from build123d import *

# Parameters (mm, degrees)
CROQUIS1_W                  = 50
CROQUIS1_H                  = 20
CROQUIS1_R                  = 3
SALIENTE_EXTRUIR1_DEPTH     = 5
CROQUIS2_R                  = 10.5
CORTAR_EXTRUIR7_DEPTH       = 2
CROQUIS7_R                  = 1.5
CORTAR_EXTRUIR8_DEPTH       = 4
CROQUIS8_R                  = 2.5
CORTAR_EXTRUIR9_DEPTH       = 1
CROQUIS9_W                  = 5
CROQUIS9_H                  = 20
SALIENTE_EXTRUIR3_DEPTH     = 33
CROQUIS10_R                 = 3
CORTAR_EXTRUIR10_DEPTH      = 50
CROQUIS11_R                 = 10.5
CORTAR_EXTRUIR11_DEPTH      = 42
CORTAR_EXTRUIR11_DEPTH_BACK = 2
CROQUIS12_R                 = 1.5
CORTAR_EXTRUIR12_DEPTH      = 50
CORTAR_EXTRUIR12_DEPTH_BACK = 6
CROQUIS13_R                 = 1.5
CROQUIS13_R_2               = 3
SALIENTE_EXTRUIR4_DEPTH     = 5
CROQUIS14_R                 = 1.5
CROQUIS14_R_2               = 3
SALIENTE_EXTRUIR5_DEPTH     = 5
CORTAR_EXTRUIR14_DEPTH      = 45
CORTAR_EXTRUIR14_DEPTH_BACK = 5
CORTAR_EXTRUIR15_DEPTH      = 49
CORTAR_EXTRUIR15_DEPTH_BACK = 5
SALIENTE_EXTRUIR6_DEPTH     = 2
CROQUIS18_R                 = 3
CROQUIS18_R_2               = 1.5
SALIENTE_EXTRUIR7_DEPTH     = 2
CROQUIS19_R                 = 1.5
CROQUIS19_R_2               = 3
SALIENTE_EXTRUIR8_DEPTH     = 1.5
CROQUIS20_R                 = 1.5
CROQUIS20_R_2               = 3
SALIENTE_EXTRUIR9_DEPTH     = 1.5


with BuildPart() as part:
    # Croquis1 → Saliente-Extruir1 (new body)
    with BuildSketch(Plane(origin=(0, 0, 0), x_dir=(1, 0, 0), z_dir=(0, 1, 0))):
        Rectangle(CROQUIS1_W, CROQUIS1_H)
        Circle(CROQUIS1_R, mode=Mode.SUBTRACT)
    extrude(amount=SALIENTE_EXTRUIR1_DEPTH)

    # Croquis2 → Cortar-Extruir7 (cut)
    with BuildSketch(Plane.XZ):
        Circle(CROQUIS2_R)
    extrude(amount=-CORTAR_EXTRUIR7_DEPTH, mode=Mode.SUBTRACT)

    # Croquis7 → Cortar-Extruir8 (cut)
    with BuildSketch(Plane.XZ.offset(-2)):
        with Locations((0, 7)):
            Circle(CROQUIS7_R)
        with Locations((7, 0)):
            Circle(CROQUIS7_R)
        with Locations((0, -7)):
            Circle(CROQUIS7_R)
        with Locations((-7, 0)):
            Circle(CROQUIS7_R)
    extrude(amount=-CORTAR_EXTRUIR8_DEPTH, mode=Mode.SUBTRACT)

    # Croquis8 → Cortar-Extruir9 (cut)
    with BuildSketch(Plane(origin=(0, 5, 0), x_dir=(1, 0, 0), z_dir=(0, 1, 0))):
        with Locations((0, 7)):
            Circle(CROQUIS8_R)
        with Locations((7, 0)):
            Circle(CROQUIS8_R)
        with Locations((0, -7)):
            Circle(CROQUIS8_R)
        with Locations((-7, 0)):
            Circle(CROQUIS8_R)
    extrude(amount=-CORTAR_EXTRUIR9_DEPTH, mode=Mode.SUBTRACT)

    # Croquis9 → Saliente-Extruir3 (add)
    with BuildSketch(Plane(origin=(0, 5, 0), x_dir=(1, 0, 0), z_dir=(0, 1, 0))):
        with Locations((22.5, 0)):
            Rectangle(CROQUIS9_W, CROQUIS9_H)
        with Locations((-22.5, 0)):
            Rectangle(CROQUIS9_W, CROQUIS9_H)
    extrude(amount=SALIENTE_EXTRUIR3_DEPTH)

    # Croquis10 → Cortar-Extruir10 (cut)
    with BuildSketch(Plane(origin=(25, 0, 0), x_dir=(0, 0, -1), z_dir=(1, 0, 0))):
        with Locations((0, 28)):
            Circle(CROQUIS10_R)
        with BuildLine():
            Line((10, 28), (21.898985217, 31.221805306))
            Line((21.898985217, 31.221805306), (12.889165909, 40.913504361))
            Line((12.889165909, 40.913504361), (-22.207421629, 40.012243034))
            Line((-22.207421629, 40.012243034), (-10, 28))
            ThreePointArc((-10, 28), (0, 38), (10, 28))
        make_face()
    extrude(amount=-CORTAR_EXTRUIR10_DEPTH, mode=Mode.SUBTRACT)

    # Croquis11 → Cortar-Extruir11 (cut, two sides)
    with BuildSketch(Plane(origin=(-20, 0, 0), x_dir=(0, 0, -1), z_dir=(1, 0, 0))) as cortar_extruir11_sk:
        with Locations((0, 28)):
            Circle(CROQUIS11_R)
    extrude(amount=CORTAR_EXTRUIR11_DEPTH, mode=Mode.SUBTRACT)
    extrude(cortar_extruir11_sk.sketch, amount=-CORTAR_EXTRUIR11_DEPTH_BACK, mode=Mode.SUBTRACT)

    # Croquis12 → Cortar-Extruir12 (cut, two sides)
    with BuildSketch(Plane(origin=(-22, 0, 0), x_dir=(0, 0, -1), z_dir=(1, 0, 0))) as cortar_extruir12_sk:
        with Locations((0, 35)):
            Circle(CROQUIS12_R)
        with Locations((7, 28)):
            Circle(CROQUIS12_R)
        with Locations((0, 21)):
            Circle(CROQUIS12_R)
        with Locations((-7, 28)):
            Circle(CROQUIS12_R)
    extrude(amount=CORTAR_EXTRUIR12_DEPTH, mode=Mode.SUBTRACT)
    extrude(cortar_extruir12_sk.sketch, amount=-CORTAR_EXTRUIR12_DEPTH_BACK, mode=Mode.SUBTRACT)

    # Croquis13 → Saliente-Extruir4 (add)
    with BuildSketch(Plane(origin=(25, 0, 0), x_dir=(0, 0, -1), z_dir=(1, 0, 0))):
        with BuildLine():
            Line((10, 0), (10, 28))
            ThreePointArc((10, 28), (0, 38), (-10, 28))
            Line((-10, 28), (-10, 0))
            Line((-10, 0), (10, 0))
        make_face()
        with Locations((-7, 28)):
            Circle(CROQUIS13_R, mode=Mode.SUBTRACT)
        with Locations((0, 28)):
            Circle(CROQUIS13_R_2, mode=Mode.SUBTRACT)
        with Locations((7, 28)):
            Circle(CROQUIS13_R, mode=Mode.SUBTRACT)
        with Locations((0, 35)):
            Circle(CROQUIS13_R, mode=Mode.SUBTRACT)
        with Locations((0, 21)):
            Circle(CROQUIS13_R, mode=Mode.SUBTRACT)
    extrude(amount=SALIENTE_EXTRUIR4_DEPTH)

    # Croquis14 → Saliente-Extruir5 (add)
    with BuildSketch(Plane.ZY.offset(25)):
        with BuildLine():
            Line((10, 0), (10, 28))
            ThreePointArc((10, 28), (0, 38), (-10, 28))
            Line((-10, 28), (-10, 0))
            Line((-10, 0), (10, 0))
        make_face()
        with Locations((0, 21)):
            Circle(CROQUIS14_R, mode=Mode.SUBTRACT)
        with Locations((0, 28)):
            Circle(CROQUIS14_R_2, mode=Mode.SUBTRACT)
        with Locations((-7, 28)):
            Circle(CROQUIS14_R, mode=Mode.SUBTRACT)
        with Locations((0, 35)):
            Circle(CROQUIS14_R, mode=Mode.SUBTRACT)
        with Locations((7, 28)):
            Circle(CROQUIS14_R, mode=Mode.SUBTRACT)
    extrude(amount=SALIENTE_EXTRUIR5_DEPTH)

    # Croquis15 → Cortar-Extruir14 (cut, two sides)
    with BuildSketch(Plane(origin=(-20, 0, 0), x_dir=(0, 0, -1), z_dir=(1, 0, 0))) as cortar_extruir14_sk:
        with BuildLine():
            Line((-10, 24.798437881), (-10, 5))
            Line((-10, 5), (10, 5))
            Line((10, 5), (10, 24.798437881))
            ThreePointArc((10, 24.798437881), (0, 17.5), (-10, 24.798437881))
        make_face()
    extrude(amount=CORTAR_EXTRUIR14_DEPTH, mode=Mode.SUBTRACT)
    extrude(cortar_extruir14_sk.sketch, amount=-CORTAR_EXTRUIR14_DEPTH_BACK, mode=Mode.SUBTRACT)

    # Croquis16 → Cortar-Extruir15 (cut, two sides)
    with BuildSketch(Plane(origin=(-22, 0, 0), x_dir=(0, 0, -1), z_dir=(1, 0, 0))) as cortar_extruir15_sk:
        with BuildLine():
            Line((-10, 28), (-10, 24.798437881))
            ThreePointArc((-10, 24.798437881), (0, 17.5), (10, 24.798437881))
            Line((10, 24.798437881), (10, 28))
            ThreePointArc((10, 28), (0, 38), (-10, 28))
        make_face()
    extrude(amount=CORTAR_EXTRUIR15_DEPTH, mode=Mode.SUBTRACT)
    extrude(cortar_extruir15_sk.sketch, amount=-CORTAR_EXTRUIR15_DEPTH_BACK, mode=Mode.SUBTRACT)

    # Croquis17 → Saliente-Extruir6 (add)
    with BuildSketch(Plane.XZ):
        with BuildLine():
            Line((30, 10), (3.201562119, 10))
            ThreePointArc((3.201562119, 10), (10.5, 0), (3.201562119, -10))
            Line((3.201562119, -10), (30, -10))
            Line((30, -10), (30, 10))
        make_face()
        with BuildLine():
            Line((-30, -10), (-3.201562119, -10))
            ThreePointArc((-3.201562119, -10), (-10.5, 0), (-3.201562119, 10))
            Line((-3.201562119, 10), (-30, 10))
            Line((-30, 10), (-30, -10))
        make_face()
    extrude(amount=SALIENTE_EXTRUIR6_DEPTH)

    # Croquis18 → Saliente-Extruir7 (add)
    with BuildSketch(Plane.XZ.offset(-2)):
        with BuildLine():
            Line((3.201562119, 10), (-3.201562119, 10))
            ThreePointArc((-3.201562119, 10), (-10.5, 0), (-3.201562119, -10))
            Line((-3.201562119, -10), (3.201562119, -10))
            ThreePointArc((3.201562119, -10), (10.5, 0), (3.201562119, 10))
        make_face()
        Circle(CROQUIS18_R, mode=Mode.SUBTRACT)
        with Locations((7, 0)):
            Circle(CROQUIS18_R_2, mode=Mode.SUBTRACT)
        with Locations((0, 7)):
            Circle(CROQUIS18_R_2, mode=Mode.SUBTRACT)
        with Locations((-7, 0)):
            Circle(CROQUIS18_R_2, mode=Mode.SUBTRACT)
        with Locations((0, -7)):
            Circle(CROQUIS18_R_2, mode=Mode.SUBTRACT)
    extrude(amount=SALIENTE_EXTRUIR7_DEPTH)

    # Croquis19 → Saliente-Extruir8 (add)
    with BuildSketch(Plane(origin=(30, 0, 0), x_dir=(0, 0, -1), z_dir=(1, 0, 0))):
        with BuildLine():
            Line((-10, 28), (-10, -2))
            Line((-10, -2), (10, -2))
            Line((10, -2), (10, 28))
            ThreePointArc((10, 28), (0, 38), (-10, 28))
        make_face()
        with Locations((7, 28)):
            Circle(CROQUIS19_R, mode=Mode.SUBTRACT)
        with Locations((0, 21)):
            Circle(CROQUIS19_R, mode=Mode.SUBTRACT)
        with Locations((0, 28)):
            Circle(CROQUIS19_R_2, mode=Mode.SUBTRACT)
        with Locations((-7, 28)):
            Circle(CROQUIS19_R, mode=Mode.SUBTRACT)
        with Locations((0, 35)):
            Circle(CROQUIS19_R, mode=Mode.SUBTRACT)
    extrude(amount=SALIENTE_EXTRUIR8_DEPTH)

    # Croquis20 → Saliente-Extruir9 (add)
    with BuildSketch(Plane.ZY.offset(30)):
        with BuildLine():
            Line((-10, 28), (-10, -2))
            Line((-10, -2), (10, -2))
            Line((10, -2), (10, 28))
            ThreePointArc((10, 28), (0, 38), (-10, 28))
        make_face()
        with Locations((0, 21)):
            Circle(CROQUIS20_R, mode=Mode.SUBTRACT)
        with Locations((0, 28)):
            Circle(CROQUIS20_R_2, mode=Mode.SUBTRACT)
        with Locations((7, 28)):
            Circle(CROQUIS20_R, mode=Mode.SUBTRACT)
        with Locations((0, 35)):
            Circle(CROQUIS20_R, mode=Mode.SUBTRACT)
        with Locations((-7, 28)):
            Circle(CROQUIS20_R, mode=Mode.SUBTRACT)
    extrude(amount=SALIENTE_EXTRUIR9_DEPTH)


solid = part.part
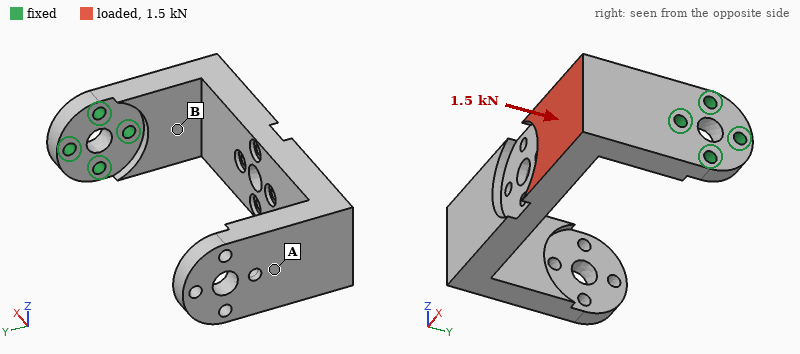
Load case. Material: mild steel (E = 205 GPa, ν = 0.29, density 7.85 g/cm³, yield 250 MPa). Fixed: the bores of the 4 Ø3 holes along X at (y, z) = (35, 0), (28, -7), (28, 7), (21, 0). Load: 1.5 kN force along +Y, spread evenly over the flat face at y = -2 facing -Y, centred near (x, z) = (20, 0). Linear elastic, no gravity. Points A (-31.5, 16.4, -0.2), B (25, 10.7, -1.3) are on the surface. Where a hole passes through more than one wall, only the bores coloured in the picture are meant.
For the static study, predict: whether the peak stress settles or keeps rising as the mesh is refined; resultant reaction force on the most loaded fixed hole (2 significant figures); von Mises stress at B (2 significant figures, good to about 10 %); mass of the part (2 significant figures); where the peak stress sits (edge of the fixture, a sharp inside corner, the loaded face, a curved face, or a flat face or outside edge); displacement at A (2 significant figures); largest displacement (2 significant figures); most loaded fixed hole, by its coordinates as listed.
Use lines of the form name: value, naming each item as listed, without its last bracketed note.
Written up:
whether the peak stress settles or keeps rising as the mesh is refined: keeps rising
resultant reaction force on the most loaded fixed hole: 1.1 kN
von Mises stress at B: 87 MPa
mass of the part: 110 g
where the peak stress sits: edge of the fixture
displacement at A: 0.24 mm
largest displacement: 0.26 mm
most loaded fixed hole, by its coordinates as listed: (21, 0)
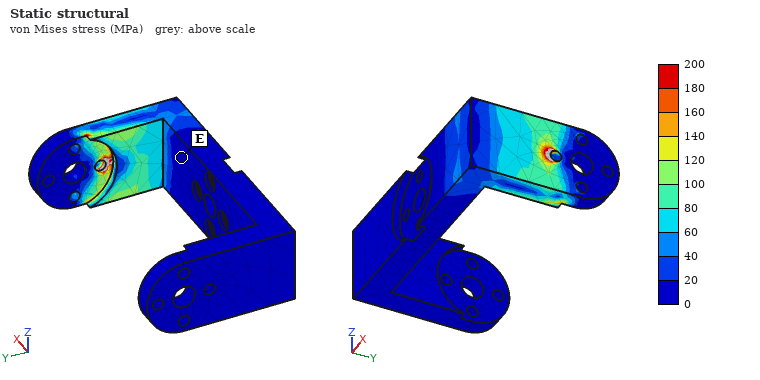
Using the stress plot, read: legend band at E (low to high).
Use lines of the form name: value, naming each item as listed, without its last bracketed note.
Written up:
legend band at E: 0 to 20 MPa
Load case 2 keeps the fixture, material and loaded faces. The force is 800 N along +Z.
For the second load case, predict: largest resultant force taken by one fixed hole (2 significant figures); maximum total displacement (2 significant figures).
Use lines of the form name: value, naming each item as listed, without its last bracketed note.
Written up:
largest resultant force taken by one fixed hole: 1.0 kN
maximum total displacement: 82 µm
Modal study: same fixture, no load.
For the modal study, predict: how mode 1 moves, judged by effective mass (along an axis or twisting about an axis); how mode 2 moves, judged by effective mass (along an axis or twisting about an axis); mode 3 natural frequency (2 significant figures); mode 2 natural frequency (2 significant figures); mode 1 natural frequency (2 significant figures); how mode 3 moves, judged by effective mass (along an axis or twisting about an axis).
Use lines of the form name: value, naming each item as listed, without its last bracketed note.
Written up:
how mode 1 moves, judged by effective mass: along Y
how mode 2 moves, judged by effective mass: along Z
mode 3 natural frequency: 2000 Hz
mode 2 natural frequency: 830 Hz
mode 1 natural frequency: 550 Hz
how mode 3 moves, judged by effective mass: along X
